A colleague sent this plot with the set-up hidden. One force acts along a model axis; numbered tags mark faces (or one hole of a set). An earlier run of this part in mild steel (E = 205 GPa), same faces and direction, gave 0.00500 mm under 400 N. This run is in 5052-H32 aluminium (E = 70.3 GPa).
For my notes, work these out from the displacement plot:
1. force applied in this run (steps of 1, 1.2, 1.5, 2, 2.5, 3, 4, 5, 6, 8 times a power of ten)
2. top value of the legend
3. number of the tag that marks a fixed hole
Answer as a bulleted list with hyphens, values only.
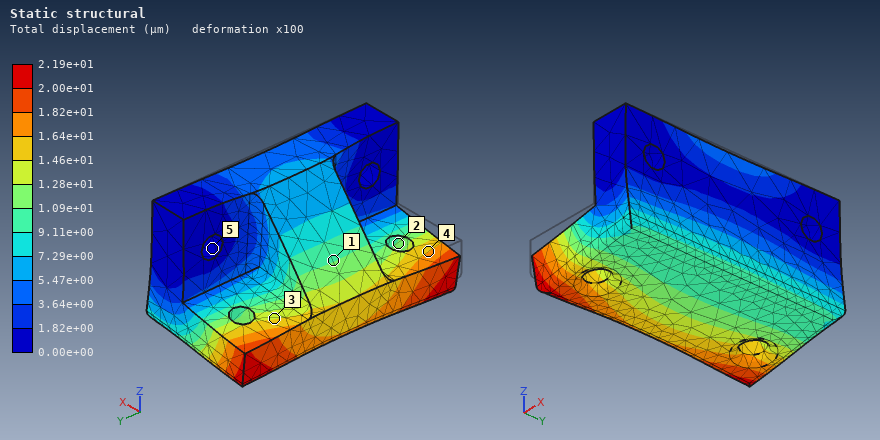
- 600 N
- 2.19e+01 µm
- 5
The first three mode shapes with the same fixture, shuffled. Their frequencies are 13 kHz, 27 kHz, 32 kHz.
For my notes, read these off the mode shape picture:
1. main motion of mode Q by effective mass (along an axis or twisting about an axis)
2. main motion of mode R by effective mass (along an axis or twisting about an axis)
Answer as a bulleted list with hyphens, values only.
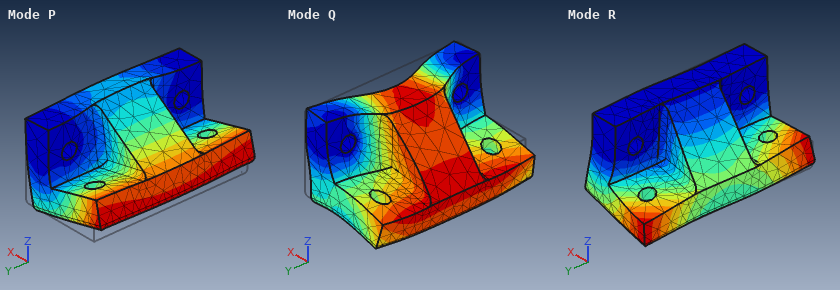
- along X
- along Y
